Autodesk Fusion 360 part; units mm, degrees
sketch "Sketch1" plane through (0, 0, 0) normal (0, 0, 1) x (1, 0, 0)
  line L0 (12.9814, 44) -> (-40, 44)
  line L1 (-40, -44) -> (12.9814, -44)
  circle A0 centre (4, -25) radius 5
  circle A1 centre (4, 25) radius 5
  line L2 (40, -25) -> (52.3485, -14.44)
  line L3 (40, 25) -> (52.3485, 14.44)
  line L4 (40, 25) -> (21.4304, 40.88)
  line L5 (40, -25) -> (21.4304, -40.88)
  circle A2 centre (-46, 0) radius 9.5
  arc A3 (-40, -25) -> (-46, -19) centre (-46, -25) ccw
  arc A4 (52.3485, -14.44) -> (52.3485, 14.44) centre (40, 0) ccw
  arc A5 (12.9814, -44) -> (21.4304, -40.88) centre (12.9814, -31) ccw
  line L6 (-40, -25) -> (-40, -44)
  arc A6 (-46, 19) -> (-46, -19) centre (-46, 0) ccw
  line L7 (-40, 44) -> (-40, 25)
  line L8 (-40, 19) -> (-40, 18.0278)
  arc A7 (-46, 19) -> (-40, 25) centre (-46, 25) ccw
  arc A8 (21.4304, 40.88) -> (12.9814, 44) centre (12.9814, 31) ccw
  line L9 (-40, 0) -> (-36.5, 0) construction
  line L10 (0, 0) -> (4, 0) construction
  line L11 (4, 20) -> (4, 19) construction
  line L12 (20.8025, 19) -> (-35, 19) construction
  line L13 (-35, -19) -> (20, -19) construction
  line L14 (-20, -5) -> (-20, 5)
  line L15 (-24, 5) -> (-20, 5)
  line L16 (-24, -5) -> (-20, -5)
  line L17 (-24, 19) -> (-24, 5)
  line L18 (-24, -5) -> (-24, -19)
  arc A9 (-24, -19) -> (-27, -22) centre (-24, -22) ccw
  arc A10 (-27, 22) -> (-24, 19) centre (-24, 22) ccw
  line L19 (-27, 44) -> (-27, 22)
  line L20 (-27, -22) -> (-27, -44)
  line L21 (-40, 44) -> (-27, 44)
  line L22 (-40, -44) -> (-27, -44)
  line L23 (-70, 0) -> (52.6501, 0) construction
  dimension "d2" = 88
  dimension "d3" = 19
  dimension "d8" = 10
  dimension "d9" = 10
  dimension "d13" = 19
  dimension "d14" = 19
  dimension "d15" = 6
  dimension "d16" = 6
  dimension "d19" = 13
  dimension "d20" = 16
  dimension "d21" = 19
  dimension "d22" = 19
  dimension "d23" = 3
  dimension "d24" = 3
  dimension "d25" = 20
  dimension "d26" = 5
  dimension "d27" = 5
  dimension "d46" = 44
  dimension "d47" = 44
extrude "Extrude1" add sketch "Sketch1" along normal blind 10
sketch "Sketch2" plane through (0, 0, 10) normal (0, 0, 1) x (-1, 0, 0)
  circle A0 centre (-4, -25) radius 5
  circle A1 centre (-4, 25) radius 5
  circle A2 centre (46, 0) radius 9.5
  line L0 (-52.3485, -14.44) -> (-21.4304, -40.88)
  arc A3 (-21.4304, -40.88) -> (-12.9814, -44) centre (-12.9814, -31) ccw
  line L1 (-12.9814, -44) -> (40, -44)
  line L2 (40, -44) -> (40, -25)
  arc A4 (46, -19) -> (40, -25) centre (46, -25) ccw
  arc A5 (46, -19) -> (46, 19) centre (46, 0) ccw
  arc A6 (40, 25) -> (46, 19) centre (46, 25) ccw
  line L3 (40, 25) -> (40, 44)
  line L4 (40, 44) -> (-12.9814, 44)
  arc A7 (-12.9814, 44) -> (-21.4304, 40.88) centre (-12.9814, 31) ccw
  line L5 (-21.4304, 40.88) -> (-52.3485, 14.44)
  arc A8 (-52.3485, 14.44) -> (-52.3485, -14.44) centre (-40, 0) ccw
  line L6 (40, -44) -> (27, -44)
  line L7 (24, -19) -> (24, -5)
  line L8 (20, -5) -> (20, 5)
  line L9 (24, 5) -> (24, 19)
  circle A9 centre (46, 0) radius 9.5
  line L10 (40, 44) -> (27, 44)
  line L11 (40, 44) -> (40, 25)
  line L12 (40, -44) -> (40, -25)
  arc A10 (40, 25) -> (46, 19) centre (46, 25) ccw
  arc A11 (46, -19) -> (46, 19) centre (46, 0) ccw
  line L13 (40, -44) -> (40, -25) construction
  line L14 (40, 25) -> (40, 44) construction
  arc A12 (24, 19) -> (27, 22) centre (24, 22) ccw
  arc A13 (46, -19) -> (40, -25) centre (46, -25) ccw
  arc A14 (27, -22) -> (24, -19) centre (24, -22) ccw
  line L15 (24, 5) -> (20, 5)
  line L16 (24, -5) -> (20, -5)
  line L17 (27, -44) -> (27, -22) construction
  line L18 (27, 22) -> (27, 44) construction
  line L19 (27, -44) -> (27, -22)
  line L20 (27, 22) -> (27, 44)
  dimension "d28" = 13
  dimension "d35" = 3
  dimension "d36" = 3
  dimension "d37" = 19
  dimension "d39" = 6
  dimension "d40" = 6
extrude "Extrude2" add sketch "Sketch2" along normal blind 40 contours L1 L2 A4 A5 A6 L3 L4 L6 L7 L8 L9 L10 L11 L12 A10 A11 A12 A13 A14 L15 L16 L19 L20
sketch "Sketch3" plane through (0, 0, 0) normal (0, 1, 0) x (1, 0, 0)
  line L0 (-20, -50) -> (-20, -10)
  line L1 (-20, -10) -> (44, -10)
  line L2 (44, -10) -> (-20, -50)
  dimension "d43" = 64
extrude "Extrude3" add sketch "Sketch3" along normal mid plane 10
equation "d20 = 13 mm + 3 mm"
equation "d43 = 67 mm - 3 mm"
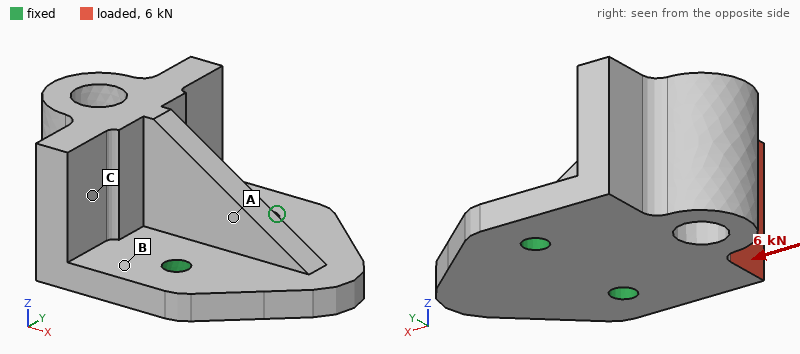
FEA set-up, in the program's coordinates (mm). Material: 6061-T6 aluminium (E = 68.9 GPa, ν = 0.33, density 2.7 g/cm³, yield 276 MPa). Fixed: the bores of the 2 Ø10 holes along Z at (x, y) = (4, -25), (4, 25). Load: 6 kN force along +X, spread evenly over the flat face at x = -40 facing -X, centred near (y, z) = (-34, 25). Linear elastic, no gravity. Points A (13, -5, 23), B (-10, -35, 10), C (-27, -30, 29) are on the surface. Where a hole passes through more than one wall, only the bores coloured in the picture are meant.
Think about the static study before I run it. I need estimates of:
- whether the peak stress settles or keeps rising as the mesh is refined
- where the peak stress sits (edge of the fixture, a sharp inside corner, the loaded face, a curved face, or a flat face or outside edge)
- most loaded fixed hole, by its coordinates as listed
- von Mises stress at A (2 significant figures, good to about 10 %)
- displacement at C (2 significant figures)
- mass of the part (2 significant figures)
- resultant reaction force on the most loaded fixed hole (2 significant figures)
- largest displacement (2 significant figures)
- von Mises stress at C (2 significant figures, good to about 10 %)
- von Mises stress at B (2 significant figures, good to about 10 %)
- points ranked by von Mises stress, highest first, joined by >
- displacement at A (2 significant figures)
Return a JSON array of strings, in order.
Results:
["keeps rising", "edge of the fixture", "(4, -25)", "13 MPa", "0.10 mm", "440 g", "6.8 kN", "0.20 mm", "26 MPa", "50 MPa", "B > C > A", "0.037 mm"]
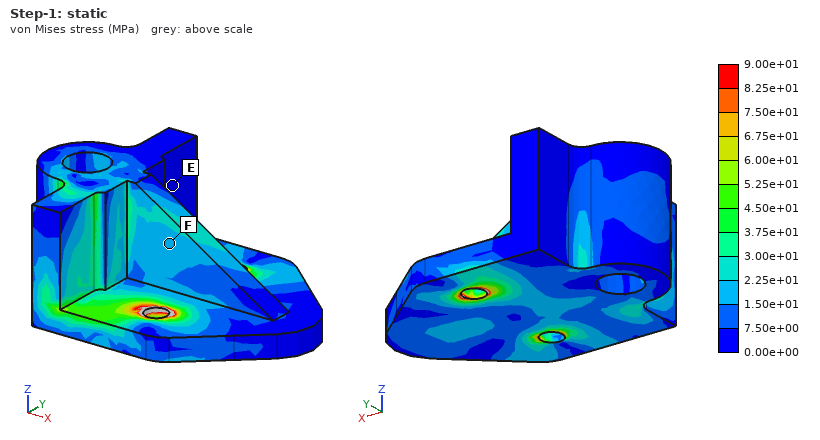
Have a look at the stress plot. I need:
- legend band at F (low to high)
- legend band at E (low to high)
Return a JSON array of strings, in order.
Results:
["1.50e+01 to 2.25e+01 MPa", "0.00e+00 to 7.50e+00 MPa"]
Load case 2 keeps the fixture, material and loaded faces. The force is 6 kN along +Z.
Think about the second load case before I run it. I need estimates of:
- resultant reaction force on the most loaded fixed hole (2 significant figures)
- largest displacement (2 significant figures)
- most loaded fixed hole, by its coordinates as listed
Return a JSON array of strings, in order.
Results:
["6.9 kN", "0.37 mm", "(4, -25)"]
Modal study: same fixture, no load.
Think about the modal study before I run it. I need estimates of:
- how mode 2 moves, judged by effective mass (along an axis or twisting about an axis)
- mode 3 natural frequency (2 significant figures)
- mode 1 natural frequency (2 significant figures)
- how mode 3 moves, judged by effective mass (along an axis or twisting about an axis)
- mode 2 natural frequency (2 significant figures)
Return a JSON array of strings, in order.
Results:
["along Y", "5400 Hz", "1600 Hz", "along Z", "2800 Hz"]
